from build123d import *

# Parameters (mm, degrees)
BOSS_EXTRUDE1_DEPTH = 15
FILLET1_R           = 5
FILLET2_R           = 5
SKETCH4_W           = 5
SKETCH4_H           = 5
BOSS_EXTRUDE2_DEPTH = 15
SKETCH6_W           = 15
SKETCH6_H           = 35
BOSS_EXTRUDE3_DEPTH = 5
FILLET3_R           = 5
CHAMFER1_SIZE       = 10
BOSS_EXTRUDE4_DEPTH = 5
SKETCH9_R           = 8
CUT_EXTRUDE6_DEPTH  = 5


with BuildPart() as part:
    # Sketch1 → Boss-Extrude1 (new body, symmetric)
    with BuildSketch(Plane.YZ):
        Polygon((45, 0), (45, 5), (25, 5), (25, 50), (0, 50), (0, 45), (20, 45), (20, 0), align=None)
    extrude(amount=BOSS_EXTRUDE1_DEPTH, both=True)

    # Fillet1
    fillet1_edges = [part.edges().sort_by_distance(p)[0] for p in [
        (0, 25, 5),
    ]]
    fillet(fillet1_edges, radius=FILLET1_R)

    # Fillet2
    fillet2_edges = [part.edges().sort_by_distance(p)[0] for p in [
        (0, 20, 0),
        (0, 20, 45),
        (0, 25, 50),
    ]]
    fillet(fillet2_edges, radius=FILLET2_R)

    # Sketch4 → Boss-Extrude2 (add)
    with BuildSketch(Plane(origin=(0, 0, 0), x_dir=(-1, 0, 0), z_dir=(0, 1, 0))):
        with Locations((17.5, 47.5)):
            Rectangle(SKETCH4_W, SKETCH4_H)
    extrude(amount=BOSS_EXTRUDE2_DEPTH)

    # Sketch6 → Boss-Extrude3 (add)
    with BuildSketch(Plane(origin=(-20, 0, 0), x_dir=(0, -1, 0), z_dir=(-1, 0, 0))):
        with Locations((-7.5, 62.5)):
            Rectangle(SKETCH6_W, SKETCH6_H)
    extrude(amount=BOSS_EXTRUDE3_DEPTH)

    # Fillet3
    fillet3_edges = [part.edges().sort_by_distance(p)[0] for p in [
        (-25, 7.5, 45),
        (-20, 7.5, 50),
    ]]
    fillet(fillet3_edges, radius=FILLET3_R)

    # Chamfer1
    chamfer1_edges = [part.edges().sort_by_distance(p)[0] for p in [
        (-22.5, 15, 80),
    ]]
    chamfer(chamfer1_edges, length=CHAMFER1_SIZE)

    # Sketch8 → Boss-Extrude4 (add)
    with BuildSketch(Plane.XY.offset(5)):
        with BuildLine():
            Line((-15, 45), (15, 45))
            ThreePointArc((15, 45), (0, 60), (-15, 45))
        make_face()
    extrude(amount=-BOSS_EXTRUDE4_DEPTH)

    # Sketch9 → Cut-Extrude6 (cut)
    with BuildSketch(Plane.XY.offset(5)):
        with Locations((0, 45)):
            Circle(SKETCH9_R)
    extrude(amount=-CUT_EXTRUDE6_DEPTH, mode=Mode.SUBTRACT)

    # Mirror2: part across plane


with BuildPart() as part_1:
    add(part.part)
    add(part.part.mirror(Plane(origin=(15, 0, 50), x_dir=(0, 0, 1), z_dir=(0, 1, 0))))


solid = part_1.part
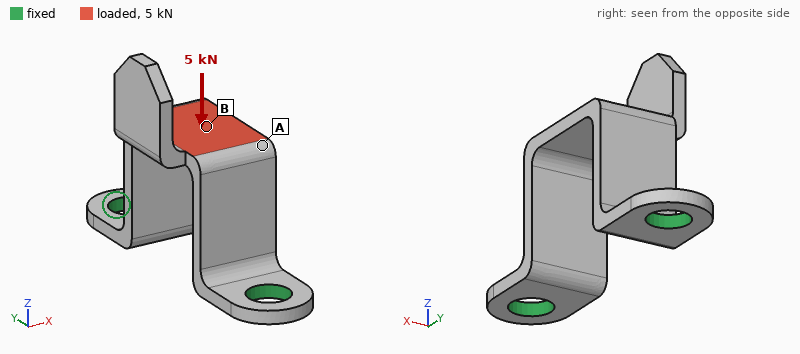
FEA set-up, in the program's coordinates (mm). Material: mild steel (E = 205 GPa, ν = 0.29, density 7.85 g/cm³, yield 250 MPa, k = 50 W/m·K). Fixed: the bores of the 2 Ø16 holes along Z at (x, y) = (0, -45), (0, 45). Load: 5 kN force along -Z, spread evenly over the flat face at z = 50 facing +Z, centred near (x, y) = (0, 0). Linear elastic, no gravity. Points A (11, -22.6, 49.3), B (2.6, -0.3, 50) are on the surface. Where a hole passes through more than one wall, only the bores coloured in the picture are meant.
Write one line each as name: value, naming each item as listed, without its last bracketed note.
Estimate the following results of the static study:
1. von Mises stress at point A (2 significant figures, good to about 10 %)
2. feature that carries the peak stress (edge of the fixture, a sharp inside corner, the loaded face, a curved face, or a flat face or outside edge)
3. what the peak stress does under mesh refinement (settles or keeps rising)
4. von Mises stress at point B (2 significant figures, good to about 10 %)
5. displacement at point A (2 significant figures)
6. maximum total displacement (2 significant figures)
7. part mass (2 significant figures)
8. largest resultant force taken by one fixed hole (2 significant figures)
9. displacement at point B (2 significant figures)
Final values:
von Mises stress at point A: 22 MPa
feature that carries the peak stress: edge of the fixture
what the peak stress does under mesh refinement: keeps rising
von Mises stress at point B: 78 MPa
displacement at point A: 26 µm
maximum total displacement: 57 µm
part mass: 270 g
largest resultant force taken by one fixed hole: 2.6 kN
displacement at point B: 51 µm
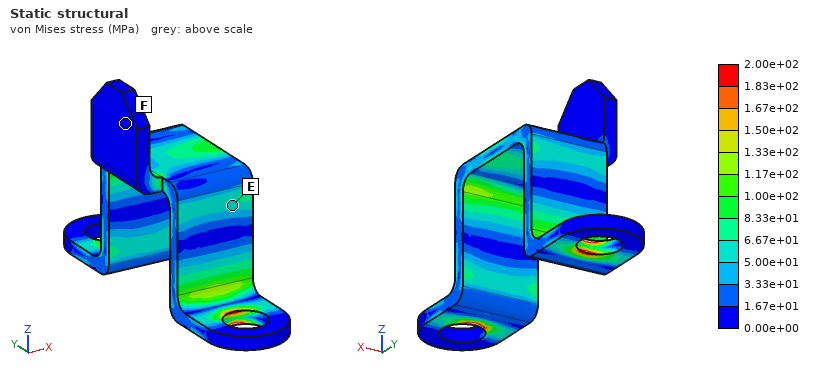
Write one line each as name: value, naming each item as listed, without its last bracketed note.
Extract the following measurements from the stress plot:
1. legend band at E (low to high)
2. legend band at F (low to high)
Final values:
legend band at E: 5.00e+01 to 6.67e+01 MPa
legend band at F: 0.00e+00 to 1.67e+01 MPa
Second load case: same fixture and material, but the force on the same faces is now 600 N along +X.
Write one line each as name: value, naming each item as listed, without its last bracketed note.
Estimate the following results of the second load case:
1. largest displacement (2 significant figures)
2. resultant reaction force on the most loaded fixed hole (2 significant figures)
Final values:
largest displacement: 0.11 mm
resultant reaction force on the most loaded fixed hole: 300 N
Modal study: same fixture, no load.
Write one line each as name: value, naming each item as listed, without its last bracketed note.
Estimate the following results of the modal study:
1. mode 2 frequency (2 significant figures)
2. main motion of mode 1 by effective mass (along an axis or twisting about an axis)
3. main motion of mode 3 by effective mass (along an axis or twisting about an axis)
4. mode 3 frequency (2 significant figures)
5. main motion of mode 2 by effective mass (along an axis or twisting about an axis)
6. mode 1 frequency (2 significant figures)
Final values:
mode 2 frequency: 1600 Hz
main motion of mode 1 by effective mass: along X
main motion of mode 3 by effective mass: twisting about Z
mode 3 frequency: 2600 Hz
main motion of mode 2 by effective mass: along Y
mode 1 frequency: 1200 Hz
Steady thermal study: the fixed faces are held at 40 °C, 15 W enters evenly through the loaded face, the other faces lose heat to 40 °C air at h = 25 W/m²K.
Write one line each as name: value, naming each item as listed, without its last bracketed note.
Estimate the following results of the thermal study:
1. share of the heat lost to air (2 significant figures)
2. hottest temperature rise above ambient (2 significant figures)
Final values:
share of the heat lost to air: 47 %
hottest temperature rise above ambient: 42 K
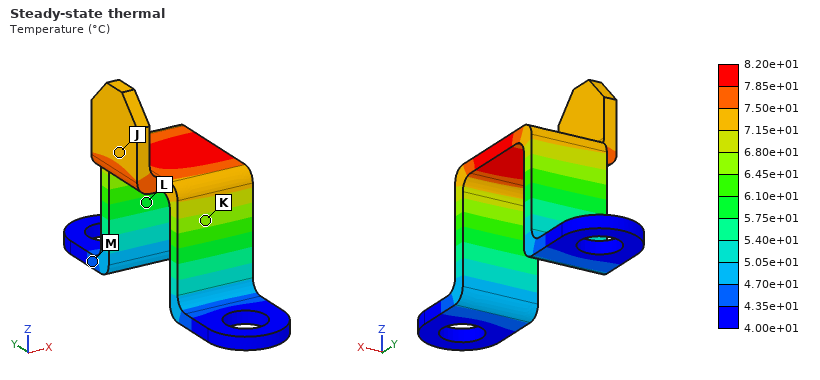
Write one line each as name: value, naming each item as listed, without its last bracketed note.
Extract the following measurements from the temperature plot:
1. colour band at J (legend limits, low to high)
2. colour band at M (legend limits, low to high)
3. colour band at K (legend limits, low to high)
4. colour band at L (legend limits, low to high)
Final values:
colour band at J: 7.15e+01 to 7.50e+01 °C
colour band at M: 4.35e+01 to 4.70e+01 °C
colour band at K: 6.45e+01 to 6.80e+01 °C
colour band at L: 5.75e+01 to 6.10e+01 °C
